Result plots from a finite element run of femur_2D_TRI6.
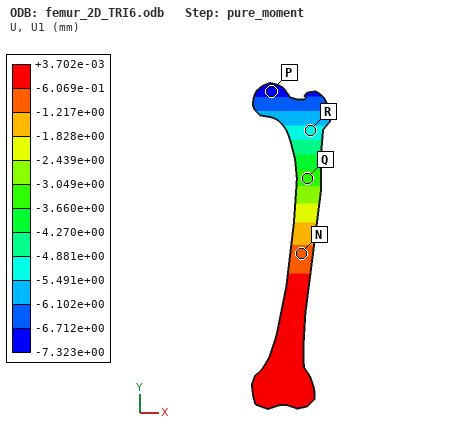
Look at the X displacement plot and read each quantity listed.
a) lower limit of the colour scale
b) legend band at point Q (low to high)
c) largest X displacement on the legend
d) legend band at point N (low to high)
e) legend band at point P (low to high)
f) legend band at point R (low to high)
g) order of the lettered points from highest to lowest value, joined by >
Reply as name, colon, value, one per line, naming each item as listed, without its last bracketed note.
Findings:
lower limit of the colour scale: -7.323e+00 mm
legend band at point Q: -3.660e+00 to -3.049e+00 mm
largest X displacement on the legend: +3.702e-03 mm
legend band at point N: -1.217e+00 to -6.069e-01 mm
legend band at point P: -7.323e+00 to -6.712e+00 mm
legend band at point R: -5.491e+00 to -4.881e+00 mm
order of the lettered points from highest to lowest value, joined by >: N > Q > R > P
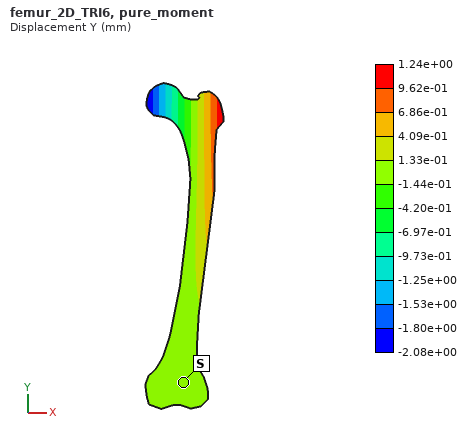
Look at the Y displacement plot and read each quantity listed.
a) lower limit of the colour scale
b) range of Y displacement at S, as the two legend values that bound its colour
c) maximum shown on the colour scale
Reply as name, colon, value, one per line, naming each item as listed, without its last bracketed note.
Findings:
lower limit of the colour scale: -2.08e+00 mm
range of Y displacement at S, as the two legend values that bound its colour: -1.44e-01 to 1.33e-01 mm
maximum shown on the colour scale: 1.24e+00 mm
